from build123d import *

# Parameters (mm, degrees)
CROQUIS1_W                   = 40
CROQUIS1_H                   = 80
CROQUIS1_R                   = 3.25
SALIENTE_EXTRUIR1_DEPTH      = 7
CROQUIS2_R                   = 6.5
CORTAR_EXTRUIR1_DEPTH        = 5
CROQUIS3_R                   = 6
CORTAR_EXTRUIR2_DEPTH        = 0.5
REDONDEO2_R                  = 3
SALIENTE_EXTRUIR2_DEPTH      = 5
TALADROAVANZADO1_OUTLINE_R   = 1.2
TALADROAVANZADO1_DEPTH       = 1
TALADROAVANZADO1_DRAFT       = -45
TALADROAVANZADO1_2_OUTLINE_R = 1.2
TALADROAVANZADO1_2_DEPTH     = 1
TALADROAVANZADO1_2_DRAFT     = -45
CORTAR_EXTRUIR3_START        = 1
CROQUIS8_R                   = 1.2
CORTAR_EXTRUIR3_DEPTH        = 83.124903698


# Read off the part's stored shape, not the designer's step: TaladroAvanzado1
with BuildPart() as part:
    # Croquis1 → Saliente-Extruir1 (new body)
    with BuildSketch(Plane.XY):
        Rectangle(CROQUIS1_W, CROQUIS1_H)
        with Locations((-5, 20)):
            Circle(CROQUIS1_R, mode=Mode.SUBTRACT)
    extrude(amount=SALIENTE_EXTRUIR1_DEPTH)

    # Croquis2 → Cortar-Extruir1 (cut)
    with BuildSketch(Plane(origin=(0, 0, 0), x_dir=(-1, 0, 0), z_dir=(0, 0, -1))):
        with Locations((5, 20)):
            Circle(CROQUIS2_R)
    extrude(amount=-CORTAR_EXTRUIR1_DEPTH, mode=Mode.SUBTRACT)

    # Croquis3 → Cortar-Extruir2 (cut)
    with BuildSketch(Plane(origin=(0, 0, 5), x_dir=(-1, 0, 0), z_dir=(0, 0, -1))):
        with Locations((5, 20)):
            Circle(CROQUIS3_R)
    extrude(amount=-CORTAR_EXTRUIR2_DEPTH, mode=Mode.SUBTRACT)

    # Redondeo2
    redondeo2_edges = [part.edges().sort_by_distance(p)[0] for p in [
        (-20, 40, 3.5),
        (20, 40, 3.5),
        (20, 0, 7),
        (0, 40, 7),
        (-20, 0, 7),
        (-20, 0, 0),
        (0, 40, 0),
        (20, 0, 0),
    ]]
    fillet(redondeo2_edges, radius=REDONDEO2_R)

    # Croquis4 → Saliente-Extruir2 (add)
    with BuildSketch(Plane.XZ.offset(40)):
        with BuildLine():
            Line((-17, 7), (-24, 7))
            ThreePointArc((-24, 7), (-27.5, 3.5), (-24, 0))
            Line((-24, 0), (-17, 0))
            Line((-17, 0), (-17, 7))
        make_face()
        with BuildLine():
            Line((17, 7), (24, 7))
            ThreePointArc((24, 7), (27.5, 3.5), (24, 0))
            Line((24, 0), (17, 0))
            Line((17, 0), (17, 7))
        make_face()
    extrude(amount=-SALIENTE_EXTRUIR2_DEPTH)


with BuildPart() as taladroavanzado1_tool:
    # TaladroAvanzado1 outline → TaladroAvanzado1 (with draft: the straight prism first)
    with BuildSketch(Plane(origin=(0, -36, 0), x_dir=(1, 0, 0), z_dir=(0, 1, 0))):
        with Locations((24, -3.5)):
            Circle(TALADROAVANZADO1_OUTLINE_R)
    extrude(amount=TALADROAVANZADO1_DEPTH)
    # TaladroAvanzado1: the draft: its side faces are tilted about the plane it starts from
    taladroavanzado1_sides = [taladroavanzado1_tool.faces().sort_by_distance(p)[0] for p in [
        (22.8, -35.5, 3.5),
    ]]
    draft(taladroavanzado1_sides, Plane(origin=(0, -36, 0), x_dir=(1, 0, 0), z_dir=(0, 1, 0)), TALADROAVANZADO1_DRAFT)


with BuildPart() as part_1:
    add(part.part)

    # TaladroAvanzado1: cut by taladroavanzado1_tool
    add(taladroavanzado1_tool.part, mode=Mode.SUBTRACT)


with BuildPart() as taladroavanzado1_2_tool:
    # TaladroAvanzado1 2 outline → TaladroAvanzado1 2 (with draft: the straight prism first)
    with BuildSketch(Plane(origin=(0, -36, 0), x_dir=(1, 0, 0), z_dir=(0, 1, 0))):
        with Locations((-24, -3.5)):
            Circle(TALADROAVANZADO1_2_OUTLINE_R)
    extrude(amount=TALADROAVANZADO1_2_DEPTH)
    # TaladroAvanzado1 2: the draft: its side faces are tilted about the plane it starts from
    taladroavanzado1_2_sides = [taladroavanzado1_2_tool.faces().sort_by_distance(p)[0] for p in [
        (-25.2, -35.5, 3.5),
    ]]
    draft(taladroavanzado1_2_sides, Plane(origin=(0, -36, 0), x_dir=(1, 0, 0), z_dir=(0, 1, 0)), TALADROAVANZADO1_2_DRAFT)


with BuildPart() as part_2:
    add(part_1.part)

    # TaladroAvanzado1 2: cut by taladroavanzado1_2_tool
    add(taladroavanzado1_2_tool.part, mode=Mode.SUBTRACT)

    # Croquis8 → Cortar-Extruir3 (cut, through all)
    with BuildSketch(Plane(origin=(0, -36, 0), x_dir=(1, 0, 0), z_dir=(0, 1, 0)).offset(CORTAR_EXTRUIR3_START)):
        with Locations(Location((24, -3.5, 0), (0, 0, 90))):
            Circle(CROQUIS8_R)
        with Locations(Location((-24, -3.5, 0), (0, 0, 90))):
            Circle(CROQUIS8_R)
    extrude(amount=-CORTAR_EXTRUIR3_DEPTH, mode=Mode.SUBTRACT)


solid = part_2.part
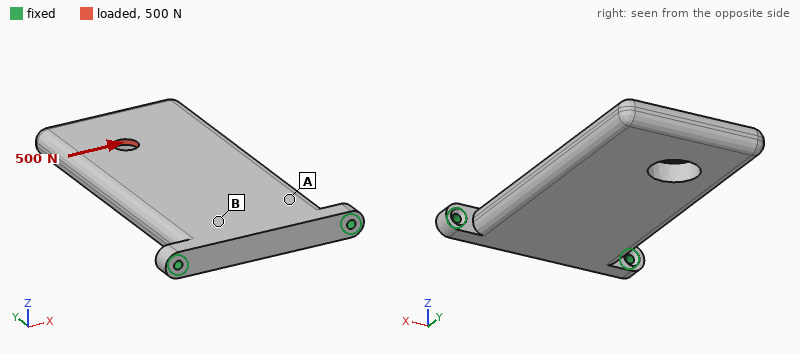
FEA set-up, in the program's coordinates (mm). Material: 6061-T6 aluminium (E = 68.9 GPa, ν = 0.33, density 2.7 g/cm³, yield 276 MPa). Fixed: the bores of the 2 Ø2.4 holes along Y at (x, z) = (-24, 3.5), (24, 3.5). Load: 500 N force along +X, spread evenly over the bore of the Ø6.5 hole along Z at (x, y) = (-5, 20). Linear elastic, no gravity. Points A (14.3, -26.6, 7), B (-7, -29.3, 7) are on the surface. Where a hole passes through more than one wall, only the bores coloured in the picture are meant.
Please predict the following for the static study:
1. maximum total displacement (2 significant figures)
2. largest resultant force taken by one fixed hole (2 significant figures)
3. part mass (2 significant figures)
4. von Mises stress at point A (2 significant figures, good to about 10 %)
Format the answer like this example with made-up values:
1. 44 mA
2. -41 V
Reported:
1. 61 µm
2. 720 N
3. 58 g
4. 13 MPa
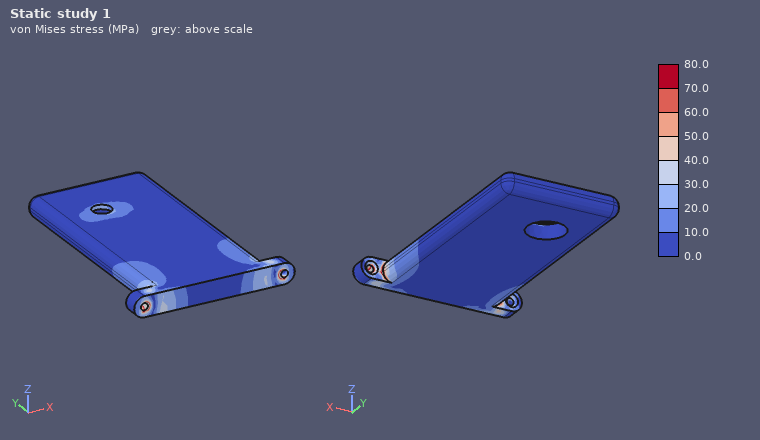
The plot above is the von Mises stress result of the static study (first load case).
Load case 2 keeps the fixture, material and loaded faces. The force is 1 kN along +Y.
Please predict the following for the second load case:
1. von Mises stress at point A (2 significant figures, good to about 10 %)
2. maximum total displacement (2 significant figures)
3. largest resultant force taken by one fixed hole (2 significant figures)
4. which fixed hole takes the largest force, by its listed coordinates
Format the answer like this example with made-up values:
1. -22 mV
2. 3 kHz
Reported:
1. 15 MPa
2. 0.28 mm
3. 680 N
4. (-24, 3.5)
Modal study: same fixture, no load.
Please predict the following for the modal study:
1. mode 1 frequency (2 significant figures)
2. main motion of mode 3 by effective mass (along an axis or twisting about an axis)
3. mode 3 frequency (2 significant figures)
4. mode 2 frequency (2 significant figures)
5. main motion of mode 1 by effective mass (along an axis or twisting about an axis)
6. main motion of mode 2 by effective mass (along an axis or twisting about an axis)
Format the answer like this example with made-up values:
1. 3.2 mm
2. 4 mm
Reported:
1. 470 Hz
2. twisting about Y
3. 3400 Hz
4. 3100 Hz
5. along Z
6. along X
